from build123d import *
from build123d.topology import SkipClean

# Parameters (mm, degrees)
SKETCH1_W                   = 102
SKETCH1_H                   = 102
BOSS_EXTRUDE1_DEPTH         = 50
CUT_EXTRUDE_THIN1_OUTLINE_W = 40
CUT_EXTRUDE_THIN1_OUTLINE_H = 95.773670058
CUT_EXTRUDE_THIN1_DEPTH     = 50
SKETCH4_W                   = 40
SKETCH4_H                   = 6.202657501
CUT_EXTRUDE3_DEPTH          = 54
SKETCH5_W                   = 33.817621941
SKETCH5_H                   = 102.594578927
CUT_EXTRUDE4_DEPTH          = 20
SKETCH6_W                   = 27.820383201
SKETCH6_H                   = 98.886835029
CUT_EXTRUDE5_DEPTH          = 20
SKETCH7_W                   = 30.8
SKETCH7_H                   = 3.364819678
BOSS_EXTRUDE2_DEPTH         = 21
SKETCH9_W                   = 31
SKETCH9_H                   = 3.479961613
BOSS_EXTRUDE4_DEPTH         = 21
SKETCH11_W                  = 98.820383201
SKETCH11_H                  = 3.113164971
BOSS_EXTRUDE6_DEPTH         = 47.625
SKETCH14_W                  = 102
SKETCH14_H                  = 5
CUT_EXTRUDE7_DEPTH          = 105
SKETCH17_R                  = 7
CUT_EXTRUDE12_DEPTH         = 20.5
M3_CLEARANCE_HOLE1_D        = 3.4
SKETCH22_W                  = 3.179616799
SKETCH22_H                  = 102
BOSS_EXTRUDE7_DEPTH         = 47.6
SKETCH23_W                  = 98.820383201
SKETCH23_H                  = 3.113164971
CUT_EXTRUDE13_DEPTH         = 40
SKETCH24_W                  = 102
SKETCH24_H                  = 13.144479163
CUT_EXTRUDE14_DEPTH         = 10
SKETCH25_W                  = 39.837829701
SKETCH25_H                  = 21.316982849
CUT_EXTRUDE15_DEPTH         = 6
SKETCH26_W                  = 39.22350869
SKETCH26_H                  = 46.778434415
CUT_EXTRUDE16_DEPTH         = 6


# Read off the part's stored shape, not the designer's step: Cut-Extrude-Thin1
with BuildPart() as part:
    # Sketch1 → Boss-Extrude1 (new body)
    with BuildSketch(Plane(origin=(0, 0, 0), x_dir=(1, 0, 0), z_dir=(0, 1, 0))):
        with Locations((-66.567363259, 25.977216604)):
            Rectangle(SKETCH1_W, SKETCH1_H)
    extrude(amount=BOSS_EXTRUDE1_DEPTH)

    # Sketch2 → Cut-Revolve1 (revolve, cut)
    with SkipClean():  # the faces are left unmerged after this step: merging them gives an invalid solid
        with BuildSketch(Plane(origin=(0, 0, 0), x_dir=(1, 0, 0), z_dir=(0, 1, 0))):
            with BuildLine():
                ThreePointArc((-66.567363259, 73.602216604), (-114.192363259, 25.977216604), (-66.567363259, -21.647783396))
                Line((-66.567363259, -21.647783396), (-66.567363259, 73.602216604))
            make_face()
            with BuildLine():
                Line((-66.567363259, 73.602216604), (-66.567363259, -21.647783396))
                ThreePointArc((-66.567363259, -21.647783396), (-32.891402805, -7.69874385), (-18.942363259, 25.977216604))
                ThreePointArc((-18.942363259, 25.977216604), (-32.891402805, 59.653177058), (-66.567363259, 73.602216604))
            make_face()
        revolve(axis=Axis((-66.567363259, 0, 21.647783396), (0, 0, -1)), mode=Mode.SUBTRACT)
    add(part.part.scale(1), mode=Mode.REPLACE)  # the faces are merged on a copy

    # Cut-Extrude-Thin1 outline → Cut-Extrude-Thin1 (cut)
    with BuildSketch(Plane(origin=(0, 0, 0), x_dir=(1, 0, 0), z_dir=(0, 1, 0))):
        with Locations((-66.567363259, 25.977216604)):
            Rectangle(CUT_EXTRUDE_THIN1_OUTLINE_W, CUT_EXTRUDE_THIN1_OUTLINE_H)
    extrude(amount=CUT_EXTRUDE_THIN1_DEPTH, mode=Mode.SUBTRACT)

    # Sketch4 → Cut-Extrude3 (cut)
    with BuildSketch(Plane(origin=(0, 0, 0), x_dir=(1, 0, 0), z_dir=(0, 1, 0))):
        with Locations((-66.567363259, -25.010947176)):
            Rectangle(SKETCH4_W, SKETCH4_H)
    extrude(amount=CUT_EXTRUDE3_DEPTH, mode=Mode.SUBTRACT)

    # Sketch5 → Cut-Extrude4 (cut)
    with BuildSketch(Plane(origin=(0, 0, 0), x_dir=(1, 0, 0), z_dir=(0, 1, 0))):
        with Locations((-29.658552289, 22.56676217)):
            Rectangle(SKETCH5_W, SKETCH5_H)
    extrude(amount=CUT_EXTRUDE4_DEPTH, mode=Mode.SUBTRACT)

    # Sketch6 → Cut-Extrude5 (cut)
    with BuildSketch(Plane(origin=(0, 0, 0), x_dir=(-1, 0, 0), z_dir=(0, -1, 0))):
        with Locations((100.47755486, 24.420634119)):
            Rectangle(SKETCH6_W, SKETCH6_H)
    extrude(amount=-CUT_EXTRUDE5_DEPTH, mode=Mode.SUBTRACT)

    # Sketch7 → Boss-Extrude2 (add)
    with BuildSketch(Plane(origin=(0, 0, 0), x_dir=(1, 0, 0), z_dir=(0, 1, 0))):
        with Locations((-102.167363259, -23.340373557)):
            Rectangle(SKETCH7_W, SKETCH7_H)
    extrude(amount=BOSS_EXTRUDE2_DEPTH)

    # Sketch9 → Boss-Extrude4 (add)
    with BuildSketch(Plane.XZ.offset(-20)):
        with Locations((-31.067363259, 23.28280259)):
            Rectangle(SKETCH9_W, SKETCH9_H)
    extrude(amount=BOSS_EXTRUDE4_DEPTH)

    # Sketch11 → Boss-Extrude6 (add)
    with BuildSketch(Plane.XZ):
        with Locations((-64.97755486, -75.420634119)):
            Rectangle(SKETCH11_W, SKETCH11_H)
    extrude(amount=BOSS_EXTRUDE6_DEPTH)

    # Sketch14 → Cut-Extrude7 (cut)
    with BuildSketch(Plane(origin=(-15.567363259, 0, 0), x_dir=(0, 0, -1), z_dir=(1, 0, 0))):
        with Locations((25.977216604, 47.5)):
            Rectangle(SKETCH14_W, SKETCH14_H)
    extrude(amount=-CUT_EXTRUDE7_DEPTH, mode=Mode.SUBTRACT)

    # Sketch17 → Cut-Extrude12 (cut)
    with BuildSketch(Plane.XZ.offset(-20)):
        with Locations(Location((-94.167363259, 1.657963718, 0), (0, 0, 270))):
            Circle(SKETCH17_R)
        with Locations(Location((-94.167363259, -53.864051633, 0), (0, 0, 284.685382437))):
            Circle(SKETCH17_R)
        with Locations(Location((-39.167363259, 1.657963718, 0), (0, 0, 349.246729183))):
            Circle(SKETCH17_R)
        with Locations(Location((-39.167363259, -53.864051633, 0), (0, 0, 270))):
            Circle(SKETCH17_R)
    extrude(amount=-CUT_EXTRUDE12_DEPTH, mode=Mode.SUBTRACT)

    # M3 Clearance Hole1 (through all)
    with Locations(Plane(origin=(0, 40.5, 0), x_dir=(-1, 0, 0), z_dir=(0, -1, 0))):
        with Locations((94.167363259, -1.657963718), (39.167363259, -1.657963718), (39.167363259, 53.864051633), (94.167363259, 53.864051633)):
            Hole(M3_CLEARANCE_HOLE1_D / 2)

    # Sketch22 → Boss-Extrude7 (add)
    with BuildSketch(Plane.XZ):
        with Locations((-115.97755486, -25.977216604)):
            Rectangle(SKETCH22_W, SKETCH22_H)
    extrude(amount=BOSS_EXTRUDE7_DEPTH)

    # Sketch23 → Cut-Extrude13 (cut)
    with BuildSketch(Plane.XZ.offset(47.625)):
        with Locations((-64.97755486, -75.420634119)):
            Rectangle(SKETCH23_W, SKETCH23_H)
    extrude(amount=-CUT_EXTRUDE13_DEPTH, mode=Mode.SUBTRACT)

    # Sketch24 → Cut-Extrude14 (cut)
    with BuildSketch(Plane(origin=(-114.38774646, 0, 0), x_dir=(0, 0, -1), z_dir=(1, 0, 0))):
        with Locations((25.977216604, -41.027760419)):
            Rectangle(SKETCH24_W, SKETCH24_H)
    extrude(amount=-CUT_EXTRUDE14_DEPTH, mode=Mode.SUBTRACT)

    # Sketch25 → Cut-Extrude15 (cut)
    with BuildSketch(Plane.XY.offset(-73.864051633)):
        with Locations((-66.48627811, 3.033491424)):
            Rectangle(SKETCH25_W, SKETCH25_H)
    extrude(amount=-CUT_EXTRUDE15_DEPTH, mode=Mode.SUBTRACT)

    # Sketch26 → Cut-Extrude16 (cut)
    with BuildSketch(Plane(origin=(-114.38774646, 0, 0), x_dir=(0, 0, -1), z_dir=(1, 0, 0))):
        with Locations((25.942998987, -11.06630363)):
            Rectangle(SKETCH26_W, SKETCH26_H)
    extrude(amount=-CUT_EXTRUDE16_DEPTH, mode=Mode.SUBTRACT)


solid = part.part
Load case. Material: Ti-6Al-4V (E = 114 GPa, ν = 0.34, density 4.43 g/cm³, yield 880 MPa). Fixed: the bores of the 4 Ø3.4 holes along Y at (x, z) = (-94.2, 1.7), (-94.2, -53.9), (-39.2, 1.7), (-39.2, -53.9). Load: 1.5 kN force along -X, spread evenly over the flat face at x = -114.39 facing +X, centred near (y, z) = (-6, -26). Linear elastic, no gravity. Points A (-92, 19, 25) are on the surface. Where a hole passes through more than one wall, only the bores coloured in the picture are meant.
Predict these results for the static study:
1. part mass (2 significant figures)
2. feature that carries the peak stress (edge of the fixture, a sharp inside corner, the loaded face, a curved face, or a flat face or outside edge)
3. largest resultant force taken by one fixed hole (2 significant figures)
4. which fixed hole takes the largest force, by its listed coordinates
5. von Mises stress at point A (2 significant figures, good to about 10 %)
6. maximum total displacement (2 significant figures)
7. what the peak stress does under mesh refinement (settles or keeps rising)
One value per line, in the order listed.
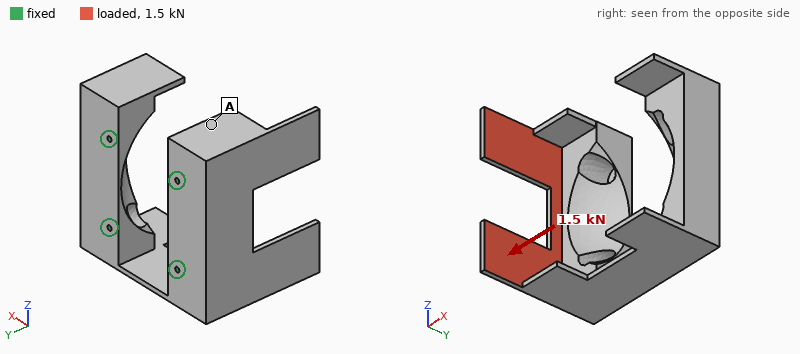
640 g
edge of the fixture
1.5 kN
(-39.2, -53.9)
38 MPa
1.00 mm
keeps rising
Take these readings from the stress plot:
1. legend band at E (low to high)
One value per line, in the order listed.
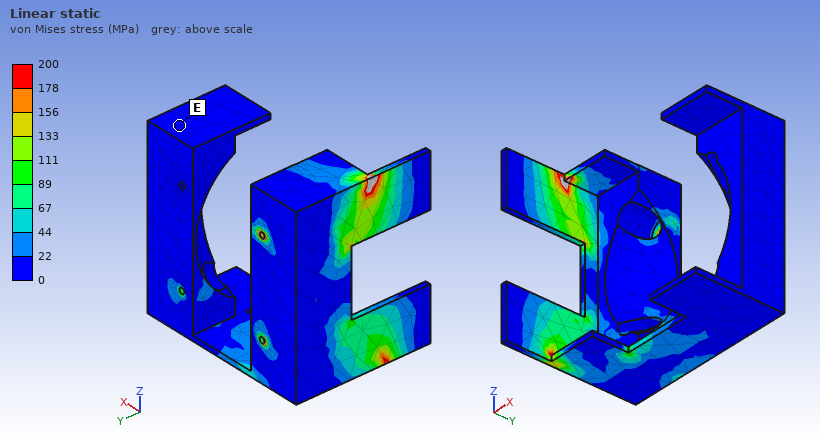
0 to 22 MPa
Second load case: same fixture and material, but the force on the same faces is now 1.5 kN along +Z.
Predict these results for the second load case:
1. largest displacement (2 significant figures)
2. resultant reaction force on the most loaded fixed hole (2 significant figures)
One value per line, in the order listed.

84 µm
1.6 kN
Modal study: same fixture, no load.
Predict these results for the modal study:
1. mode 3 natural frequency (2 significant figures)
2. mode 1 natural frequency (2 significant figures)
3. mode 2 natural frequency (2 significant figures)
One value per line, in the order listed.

2400 Hz
1200 Hz
1500 Hz
